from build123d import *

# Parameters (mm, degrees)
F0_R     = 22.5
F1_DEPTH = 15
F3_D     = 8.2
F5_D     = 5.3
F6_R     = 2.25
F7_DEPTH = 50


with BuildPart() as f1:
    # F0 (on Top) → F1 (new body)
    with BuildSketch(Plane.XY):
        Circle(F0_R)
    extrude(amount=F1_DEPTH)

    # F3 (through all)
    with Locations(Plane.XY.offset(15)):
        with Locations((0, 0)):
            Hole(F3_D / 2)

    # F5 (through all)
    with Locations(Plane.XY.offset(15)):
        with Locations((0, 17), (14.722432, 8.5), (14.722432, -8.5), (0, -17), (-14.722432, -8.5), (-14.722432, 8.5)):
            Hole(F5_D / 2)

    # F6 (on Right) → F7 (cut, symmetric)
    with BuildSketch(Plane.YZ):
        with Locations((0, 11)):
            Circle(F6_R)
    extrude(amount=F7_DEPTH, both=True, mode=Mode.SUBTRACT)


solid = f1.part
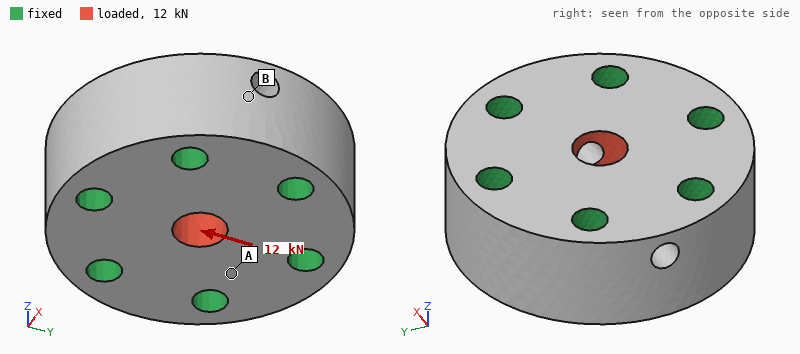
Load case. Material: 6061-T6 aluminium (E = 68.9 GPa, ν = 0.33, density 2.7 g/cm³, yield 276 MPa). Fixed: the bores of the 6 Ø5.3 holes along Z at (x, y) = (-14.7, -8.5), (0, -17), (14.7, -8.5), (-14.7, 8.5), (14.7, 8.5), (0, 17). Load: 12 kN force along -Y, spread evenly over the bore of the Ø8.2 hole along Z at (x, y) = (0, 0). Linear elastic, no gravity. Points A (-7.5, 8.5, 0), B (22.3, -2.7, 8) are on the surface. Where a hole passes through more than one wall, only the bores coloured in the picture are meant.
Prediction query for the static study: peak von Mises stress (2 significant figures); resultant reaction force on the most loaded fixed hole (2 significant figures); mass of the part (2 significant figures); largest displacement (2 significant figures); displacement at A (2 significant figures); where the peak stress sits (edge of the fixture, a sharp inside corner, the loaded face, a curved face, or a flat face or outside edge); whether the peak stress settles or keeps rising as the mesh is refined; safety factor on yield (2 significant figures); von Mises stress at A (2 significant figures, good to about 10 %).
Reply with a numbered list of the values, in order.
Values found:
1. 82 MPa
2. 3.5 kN
3. 55 g
4. 4.8 µm
5. 1.6 µm
6. the loaded face
7. settles
8. 3.4
9. 12 MPa
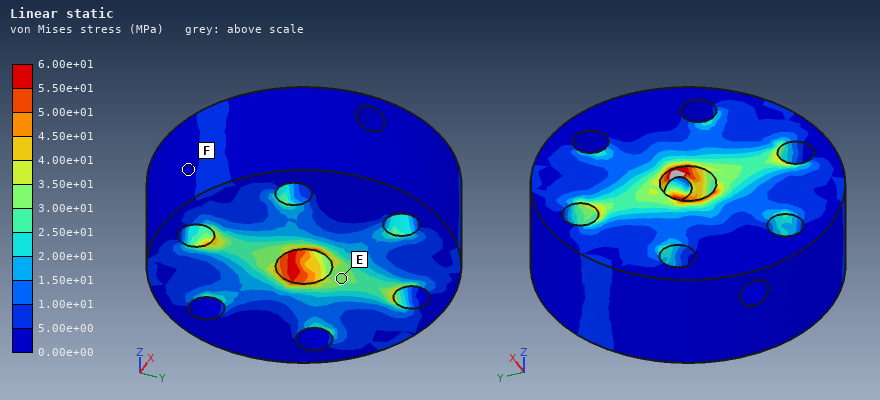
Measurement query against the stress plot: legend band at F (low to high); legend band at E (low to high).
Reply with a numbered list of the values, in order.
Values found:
1. 0.00e+00 to 5.00e+00 MPa
2. 3.00e+01 to 3.50e+01 MPa
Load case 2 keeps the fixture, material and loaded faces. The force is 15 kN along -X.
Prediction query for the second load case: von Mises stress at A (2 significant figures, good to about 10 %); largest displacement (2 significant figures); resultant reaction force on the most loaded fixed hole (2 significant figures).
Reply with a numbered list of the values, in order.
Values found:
1. 17 MPa
2. 6.0 µm
3. 3.6 kN
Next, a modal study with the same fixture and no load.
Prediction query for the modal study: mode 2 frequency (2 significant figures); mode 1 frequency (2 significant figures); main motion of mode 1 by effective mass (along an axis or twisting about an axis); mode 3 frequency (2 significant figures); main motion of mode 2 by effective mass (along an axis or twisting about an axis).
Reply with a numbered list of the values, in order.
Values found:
1. 83 kHz
2. 64 kHz
3. along Z
4. 87 kHz
5. twisting about X
